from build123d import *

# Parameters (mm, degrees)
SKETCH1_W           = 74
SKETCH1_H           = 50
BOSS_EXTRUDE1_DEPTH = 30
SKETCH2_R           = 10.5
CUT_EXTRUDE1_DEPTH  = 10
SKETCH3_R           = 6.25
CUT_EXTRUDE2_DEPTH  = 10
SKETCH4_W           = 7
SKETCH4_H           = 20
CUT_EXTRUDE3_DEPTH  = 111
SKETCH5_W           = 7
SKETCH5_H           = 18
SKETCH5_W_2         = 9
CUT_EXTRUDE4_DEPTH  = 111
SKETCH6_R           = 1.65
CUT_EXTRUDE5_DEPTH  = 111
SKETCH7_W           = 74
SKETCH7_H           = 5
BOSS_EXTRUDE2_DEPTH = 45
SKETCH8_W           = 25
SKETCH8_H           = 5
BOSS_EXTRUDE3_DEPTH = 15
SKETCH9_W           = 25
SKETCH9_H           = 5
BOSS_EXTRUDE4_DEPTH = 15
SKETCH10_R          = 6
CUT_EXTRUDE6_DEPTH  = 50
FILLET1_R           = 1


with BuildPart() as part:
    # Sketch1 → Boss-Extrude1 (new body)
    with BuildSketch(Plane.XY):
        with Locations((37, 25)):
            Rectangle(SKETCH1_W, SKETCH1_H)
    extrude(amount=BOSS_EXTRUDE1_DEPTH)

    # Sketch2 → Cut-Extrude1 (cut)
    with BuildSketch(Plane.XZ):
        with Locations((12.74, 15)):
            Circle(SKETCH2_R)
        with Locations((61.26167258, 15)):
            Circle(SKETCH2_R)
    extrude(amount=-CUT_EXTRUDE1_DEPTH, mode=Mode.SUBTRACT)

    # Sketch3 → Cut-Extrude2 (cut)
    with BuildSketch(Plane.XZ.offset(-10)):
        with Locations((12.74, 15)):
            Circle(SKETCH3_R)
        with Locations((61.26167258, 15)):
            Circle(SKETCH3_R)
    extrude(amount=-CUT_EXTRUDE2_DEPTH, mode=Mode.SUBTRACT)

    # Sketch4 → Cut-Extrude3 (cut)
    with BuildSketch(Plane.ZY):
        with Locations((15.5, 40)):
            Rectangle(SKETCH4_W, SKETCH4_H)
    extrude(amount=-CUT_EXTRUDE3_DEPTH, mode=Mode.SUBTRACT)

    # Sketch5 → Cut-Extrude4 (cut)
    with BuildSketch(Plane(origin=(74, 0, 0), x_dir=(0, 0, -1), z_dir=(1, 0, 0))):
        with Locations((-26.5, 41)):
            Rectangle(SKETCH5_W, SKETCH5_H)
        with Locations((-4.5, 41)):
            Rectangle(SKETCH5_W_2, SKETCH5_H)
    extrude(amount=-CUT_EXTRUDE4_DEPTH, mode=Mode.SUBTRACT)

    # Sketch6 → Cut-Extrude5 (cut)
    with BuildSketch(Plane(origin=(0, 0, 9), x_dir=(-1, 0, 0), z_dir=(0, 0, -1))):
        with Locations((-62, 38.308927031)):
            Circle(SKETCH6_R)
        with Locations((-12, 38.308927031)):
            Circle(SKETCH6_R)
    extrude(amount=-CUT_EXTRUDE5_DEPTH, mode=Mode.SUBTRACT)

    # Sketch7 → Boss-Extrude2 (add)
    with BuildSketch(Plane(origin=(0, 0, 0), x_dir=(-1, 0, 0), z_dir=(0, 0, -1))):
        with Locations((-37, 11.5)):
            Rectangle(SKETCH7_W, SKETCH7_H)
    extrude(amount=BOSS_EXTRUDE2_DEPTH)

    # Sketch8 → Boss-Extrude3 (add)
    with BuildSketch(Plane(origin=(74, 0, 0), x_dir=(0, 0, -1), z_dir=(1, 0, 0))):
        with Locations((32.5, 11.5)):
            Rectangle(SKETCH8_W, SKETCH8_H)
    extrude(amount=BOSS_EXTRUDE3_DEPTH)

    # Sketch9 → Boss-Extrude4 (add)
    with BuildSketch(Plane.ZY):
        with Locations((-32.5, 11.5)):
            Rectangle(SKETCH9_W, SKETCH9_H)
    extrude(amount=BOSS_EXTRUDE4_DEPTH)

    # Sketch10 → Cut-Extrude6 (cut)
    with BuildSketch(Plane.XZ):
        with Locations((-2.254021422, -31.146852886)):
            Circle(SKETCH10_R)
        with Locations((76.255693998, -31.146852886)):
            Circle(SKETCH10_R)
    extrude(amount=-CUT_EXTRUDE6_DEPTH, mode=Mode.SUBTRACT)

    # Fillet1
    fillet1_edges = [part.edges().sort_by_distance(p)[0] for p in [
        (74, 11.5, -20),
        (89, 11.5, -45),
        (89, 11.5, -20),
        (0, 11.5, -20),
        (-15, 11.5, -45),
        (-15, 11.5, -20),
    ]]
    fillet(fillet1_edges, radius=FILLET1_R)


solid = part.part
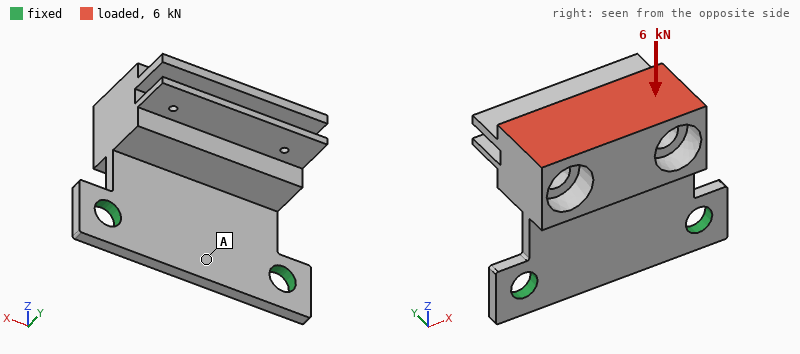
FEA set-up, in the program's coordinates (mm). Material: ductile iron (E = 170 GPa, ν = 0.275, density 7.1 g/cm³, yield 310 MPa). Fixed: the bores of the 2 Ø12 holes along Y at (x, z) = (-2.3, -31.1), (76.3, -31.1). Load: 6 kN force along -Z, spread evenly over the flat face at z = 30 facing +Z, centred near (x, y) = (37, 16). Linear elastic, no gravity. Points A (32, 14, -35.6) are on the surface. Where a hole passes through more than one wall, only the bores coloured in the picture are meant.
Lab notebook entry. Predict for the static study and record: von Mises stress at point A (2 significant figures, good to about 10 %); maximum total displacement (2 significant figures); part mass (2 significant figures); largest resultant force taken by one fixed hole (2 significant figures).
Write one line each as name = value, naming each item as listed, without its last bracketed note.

von Mises stress at point A = 21 MPa
maximum total displacement = 0.38 mm
part mass = 630 g
largest resultant force taken by one fixed hole = 3.2 kN
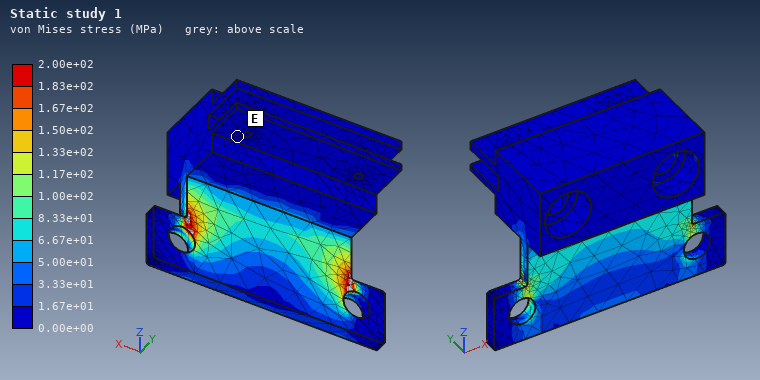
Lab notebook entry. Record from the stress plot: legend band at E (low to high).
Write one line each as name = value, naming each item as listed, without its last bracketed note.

legend band at E = 0.00e+00 to 1.67e+01 MPa
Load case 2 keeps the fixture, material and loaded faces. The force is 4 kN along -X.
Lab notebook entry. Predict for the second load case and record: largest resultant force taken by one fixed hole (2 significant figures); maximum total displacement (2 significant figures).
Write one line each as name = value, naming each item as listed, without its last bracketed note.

largest resultant force taken by one fixed hole = 3.9 kN
maximum total displacement = 38 µm
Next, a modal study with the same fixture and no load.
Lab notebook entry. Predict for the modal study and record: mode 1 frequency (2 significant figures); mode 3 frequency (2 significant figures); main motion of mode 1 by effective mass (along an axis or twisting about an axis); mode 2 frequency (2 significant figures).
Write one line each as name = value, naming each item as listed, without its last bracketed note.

mode 1 frequency = 390 Hz
mode 3 frequency = 2500 Hz
main motion of mode 1 by effective mass = along Y
mode 2 frequency = 1600 Hz
